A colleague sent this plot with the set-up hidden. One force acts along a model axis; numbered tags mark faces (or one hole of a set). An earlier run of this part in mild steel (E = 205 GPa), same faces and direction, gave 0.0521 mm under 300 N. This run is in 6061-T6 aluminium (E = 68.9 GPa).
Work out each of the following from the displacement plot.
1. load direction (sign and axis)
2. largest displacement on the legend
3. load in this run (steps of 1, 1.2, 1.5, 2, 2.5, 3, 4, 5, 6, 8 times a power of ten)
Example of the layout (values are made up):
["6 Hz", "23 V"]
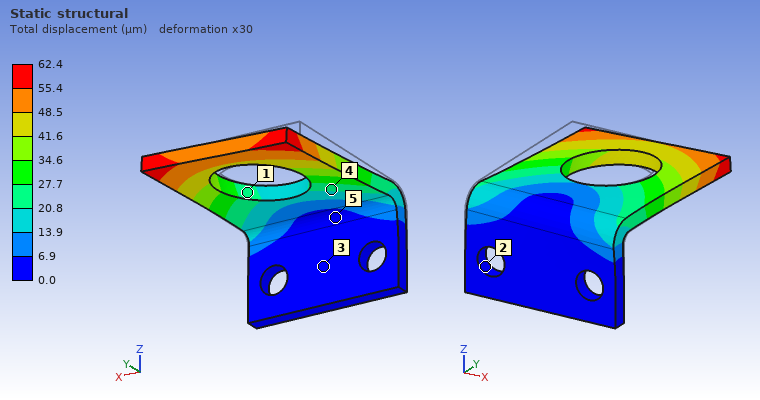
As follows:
["+X", "62.4 µm", "120 N"]
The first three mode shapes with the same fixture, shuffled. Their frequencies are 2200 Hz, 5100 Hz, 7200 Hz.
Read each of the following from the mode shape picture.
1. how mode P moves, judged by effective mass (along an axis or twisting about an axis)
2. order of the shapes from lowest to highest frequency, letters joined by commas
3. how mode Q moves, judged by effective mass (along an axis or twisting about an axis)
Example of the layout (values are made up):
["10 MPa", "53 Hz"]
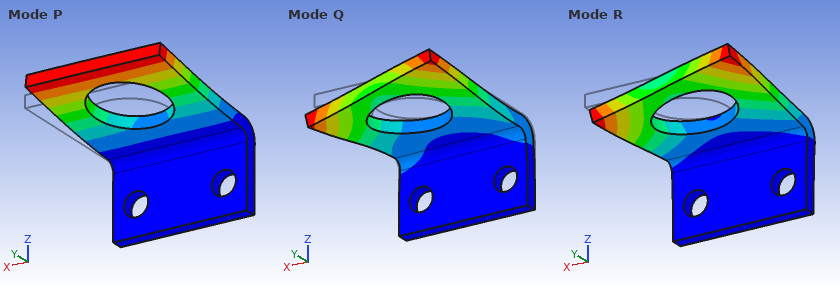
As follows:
["along Z", "P, R, Q", "along X"]
